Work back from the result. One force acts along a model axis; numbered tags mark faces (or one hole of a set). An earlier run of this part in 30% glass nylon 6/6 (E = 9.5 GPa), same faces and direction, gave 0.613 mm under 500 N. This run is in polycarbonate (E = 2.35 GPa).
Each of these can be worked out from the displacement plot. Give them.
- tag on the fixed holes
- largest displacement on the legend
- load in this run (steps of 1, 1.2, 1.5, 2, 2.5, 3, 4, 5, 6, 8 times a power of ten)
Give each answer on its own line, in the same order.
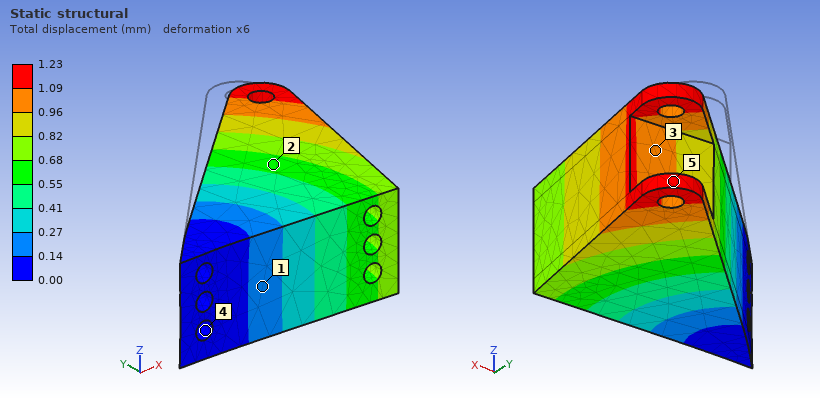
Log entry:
4
1.23 mm
250 N
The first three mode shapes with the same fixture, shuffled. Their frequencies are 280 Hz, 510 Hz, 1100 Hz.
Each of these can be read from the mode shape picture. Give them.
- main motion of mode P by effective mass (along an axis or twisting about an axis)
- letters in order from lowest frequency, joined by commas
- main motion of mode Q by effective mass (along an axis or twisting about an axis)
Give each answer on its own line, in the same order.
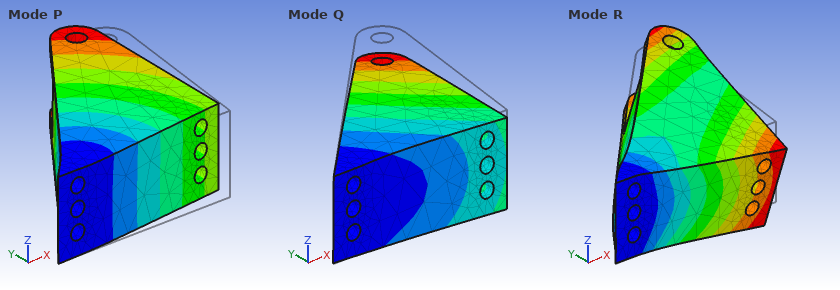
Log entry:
along Y
P, Q, R
along Z
